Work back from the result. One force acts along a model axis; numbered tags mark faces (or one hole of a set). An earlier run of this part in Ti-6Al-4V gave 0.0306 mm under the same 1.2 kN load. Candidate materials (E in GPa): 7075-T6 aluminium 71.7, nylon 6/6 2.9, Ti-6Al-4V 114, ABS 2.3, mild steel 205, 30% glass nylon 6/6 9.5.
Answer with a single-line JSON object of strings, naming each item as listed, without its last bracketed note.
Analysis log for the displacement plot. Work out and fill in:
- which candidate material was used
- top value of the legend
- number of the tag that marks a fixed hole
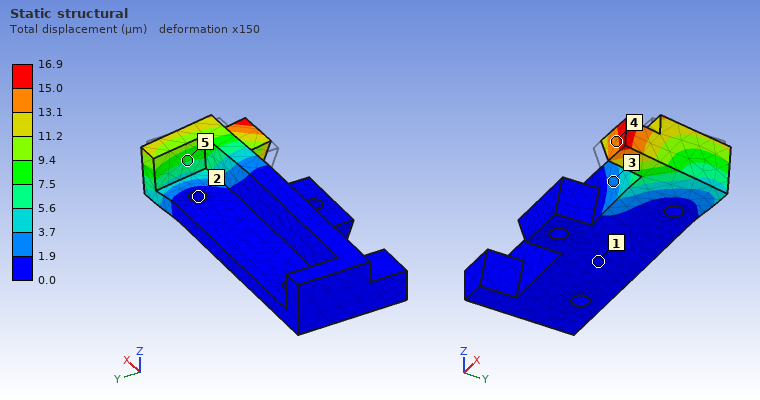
{"which candidate material was used": "mild steel", "top value of the legend": "16.9 µm", "number of the tag that marks a fixed hole": "2"}
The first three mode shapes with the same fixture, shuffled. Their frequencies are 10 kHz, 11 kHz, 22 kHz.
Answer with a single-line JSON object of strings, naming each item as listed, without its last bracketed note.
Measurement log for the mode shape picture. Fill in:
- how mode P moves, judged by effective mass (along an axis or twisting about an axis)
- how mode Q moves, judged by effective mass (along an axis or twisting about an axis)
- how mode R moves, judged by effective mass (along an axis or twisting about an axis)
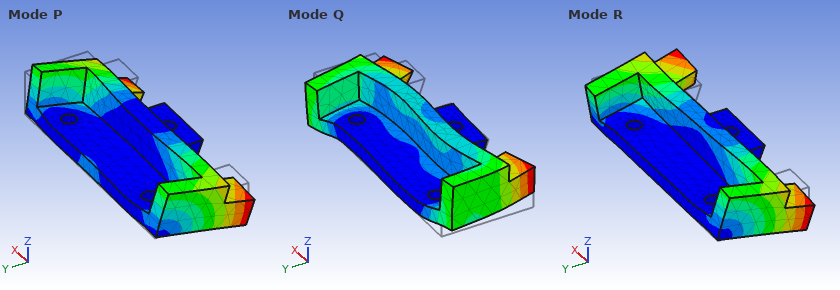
{"how mode P moves, judged by effective mass": "along Z", "how mode Q moves, judged by effective mass": "along X", "how mode R moves, judged by effective mass": "twisting about Y"}
